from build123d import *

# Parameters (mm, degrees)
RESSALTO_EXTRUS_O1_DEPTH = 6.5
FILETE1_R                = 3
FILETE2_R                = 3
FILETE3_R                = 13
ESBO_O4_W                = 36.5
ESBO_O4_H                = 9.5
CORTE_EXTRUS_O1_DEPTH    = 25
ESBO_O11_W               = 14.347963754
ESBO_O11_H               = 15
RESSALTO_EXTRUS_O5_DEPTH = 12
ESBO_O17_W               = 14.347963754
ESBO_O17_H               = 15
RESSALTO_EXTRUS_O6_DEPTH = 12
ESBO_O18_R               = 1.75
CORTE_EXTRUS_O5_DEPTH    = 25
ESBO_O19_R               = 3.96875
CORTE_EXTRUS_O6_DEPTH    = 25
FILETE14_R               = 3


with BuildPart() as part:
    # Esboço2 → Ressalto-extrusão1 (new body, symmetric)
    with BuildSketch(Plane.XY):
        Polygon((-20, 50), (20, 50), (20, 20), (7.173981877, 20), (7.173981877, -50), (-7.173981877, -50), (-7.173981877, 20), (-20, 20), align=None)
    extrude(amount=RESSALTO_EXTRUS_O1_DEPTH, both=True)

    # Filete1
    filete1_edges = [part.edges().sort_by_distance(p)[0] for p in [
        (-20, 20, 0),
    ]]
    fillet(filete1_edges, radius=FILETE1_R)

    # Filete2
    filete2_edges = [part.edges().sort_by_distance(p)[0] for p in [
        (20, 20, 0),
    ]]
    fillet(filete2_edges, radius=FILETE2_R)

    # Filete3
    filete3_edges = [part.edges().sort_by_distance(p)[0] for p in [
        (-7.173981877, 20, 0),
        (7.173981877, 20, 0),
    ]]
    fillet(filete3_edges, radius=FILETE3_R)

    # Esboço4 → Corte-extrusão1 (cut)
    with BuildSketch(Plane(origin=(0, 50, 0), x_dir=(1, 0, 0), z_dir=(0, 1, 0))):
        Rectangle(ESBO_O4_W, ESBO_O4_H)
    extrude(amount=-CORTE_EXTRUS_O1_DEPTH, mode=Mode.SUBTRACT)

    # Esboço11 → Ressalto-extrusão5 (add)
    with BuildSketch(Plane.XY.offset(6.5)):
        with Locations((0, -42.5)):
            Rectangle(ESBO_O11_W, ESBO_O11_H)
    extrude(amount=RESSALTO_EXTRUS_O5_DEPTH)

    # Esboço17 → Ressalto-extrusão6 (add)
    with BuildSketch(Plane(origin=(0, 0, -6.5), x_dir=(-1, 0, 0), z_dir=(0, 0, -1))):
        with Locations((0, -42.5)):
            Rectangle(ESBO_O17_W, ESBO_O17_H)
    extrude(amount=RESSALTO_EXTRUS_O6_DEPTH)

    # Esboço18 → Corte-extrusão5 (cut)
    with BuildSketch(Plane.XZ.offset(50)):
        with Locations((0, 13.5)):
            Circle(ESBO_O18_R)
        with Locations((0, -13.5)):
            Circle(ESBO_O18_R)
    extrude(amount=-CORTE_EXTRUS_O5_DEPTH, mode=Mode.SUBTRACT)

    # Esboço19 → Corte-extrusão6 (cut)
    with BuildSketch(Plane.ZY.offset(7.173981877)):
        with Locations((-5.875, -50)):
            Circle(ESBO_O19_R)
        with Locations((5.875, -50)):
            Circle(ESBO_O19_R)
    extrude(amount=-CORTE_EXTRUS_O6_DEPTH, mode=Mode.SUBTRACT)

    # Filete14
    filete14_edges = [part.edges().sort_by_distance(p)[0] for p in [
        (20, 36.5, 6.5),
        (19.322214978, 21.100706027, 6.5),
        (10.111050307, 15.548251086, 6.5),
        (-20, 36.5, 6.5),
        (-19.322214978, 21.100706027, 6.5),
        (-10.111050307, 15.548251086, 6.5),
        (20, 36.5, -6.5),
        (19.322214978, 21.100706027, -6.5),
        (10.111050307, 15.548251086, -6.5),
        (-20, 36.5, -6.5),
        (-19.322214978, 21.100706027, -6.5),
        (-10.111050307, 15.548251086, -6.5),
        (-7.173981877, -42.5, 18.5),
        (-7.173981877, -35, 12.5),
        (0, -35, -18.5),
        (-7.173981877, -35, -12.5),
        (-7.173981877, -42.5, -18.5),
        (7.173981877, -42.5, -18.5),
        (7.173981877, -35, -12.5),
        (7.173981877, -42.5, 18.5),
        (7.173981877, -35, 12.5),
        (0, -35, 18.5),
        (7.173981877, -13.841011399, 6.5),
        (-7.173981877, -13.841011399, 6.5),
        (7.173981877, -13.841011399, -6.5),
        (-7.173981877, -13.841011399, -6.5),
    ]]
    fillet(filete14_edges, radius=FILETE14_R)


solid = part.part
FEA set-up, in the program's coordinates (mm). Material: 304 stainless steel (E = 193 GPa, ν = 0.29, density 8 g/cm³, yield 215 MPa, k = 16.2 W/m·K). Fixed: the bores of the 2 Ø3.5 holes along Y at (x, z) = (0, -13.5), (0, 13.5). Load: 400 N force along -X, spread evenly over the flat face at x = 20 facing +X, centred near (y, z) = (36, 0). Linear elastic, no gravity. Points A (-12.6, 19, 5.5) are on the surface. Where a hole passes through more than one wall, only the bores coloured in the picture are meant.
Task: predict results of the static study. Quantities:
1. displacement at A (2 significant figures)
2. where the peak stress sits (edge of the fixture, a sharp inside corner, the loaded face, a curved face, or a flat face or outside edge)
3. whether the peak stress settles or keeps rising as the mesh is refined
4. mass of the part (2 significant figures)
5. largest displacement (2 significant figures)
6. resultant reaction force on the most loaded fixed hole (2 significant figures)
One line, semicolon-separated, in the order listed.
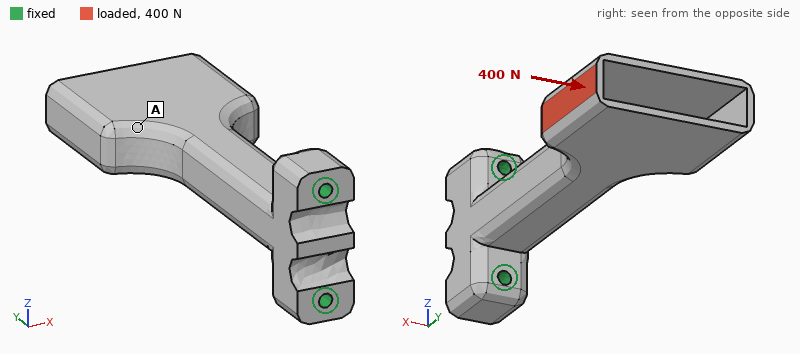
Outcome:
0.10 mm; edge of the fixture; keeps rising; 190 g; 0.18 mm; 200 N
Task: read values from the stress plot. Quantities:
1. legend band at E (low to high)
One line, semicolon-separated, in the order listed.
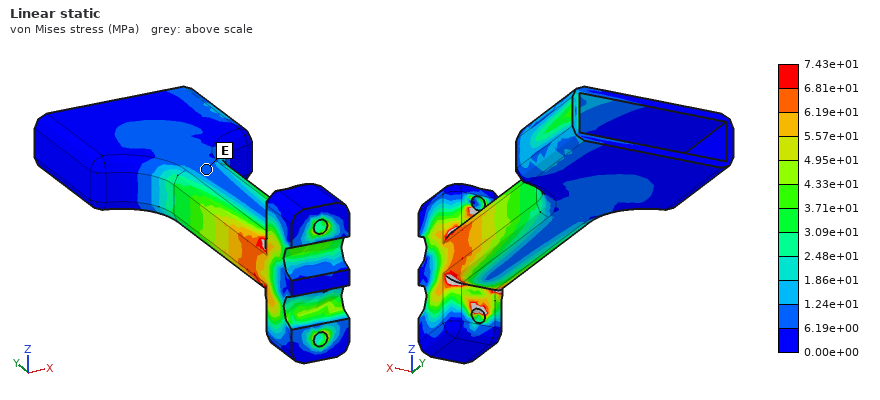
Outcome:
6.19e+00 to 1.24e+01 MPa
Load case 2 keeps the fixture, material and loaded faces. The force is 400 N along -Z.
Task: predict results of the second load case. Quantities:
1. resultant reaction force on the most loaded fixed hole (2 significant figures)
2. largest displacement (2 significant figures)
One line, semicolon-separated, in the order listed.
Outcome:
1.5 kN; 0.20 mm
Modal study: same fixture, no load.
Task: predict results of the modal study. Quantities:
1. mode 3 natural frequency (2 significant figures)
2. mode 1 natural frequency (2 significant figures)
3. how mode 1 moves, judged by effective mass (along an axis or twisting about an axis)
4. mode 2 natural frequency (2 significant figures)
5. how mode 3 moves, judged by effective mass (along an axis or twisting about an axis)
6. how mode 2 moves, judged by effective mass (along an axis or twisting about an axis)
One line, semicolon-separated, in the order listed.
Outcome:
3600 Hz; 1100 Hz; along X; 1100 Hz; twisting about Y; along Z
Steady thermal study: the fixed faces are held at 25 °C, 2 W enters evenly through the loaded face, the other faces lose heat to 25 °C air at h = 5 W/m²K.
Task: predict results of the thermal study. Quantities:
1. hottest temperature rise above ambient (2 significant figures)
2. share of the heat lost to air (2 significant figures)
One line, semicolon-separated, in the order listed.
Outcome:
46 K; 49 %
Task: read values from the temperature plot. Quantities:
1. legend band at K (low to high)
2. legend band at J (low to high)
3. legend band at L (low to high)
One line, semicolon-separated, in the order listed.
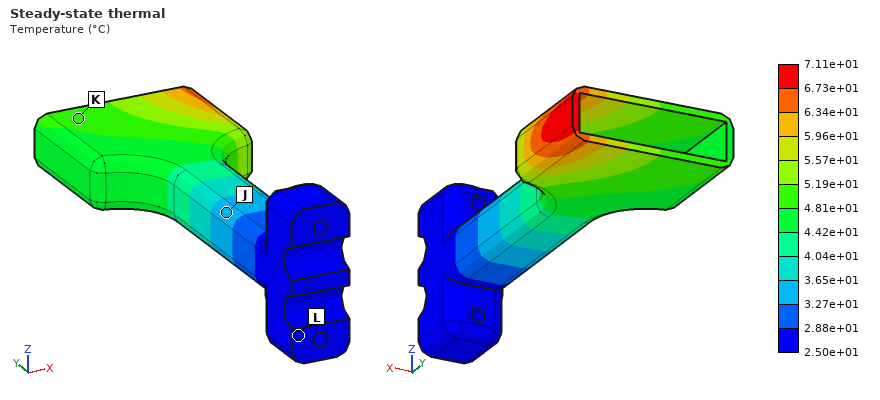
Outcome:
4.81e+01 to 5.19e+01 °C; 3.27e+01 to 3.65e+01 °C; 2.50e+01 to 2.88e+01 °C
